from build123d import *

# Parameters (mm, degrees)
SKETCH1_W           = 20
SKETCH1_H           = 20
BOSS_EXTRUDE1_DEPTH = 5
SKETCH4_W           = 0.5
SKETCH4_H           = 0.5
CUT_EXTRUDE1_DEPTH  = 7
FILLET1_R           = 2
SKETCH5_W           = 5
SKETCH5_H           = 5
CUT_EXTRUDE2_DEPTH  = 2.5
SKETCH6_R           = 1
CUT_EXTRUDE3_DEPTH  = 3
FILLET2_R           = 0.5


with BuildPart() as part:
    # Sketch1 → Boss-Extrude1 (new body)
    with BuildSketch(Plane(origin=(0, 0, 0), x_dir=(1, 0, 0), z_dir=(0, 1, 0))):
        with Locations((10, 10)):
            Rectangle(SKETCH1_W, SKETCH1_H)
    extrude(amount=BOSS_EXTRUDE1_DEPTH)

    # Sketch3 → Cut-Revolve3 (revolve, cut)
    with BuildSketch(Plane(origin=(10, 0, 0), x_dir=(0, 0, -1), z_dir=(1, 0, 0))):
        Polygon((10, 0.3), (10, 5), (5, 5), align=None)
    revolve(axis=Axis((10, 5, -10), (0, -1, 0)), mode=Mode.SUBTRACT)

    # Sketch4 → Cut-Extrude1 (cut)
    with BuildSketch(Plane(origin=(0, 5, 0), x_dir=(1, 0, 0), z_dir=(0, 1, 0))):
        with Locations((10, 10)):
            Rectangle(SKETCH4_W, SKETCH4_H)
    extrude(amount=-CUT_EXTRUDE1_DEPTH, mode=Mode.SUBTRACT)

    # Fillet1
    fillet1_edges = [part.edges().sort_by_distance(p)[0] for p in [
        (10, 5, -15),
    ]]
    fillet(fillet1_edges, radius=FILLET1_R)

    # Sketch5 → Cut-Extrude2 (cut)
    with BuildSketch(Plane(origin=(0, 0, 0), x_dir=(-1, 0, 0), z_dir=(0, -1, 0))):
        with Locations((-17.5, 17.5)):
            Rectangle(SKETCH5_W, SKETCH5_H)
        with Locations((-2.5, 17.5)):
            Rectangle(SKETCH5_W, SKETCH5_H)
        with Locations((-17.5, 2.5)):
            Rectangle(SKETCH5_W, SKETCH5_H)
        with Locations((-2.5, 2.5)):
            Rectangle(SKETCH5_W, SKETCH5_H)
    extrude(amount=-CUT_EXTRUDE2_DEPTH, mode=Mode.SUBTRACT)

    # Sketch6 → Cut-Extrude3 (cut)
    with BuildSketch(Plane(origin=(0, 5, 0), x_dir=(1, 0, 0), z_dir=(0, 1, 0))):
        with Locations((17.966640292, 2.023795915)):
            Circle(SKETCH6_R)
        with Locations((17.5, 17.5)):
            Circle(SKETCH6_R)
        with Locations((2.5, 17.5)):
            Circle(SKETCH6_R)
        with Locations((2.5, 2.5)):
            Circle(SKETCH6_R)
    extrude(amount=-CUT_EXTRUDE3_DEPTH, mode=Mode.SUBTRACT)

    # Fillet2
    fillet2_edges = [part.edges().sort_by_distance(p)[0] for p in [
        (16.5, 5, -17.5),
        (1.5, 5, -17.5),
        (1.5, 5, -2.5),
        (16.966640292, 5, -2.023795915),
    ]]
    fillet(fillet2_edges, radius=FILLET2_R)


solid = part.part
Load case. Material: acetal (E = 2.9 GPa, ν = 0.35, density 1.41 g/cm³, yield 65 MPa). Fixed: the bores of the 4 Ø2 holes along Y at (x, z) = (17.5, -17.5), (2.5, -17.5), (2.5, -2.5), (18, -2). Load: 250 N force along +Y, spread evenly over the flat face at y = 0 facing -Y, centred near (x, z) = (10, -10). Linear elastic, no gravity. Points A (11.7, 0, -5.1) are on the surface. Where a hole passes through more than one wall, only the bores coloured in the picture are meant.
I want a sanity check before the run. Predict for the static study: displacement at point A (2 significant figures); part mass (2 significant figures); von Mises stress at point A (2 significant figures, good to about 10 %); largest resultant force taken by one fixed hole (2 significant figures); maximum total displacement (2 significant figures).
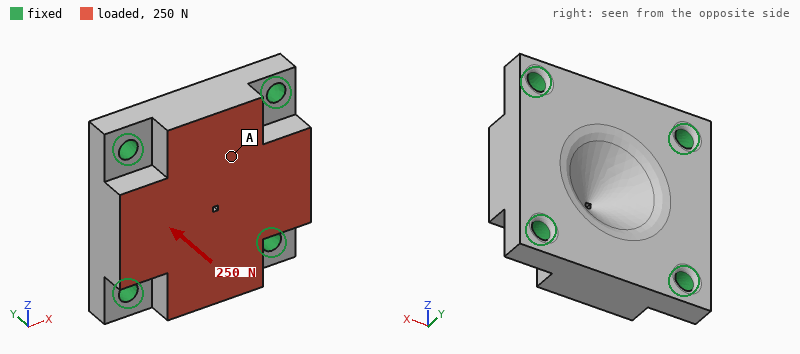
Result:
28 µm
2.2 g
2.5 MPa
73 N
35 µm
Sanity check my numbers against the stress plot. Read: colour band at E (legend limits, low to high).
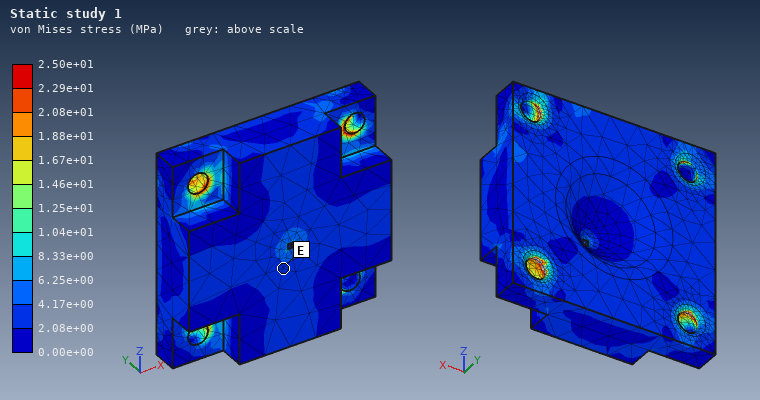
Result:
2.08e+00 to 4.17e+00 MPa
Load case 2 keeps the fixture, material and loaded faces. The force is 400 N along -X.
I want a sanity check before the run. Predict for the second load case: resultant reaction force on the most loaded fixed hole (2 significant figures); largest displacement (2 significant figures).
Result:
120 N
41 µm
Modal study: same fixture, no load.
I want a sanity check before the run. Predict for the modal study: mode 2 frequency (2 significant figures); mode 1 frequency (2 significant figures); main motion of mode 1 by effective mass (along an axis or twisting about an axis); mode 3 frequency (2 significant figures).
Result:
15 kHz
12 kHz
along Y
16 kHz
